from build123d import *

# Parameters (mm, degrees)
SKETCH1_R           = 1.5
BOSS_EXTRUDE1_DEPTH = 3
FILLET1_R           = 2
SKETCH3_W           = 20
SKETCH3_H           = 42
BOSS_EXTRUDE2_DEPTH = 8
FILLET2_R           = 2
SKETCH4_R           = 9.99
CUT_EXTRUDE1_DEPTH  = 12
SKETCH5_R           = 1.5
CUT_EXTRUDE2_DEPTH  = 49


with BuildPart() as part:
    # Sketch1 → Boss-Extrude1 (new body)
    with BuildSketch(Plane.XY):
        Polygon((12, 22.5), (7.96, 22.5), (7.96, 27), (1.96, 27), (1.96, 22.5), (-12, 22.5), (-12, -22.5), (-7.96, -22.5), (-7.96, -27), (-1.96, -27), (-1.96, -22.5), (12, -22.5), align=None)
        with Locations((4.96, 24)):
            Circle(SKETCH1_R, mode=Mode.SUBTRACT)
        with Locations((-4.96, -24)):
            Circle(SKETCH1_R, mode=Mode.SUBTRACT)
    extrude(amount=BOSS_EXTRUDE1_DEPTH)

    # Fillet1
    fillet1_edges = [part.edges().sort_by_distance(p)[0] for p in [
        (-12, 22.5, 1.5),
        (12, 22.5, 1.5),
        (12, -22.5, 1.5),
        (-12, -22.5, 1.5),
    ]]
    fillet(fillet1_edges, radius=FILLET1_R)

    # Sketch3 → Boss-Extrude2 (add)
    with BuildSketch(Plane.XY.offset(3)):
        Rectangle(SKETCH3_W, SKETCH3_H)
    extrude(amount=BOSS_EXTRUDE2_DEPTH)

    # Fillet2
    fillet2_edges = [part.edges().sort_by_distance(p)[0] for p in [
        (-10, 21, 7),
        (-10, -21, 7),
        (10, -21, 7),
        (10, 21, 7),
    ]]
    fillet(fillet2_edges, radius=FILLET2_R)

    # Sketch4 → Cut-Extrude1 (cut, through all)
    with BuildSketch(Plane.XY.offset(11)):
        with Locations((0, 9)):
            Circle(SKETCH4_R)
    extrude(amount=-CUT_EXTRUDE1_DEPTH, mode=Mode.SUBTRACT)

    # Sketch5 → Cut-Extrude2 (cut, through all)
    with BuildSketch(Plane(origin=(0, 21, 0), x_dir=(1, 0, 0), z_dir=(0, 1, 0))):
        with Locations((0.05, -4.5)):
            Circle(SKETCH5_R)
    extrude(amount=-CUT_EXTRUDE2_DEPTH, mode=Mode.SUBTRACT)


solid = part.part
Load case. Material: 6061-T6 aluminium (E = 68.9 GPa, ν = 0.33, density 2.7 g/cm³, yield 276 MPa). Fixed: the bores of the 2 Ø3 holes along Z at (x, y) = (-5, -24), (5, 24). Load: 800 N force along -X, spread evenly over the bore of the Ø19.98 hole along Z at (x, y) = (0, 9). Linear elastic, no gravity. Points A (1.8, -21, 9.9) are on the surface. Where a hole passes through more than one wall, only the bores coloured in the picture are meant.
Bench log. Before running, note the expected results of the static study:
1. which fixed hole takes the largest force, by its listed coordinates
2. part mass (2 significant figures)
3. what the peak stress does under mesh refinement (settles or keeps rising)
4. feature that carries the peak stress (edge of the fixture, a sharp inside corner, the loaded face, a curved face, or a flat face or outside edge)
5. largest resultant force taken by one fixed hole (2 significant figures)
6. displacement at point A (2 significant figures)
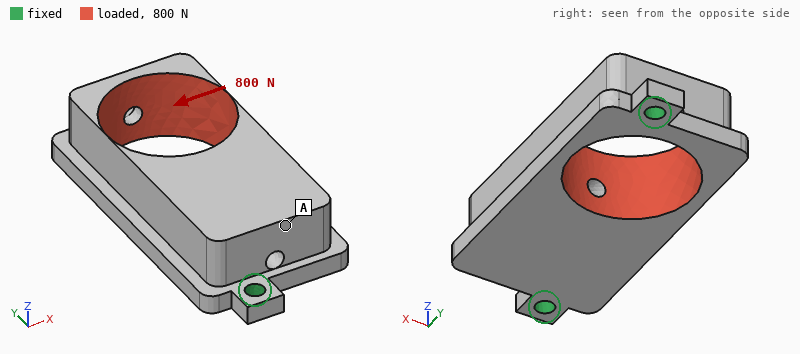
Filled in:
(5, 24)
17 g
keeps rising
edge of the fixture
530 N
35 µm
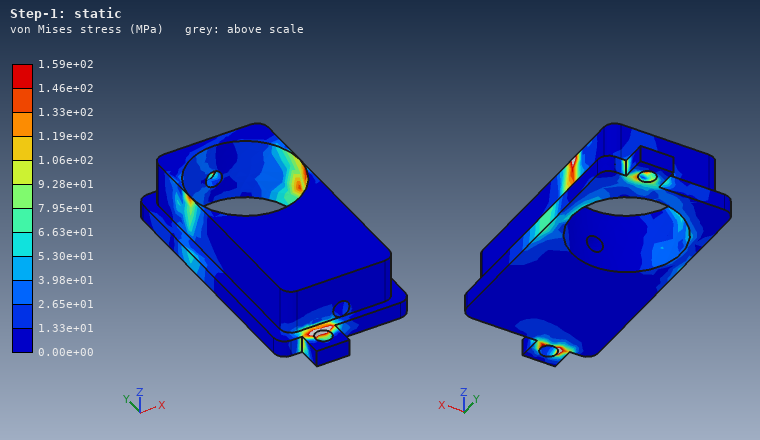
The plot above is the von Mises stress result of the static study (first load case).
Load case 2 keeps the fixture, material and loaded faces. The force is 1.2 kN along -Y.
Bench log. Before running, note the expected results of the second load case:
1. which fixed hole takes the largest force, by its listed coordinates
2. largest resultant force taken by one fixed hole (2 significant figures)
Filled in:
(-5, -24)
720 N
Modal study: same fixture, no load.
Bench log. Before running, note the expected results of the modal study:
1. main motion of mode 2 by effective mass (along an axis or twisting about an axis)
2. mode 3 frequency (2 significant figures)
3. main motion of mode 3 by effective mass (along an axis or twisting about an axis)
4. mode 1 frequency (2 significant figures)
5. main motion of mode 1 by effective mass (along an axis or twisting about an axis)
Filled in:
along Z
8300 Hz
along X
4100 Hz
along X
